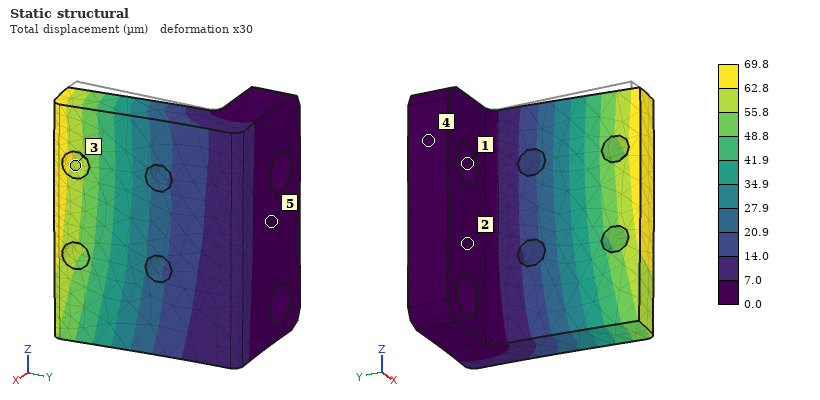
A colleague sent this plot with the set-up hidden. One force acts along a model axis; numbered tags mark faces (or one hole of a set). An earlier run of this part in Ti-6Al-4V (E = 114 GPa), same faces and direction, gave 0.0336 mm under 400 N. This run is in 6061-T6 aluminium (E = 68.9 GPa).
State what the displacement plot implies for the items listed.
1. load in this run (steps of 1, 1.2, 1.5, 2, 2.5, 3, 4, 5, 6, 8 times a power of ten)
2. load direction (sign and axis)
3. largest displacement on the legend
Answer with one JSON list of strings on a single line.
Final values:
["500 N", "+X", "69.8 µm"]
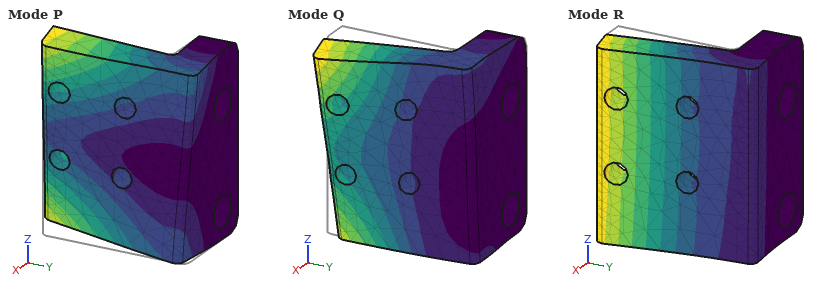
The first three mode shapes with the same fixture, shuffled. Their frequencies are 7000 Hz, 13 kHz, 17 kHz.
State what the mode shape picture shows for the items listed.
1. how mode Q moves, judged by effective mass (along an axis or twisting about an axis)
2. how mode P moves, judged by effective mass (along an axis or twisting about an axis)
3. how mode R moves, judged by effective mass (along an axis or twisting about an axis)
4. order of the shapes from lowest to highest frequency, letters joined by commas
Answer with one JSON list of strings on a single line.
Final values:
["along Z", "along Z", "along X", "R, P, Q"]
